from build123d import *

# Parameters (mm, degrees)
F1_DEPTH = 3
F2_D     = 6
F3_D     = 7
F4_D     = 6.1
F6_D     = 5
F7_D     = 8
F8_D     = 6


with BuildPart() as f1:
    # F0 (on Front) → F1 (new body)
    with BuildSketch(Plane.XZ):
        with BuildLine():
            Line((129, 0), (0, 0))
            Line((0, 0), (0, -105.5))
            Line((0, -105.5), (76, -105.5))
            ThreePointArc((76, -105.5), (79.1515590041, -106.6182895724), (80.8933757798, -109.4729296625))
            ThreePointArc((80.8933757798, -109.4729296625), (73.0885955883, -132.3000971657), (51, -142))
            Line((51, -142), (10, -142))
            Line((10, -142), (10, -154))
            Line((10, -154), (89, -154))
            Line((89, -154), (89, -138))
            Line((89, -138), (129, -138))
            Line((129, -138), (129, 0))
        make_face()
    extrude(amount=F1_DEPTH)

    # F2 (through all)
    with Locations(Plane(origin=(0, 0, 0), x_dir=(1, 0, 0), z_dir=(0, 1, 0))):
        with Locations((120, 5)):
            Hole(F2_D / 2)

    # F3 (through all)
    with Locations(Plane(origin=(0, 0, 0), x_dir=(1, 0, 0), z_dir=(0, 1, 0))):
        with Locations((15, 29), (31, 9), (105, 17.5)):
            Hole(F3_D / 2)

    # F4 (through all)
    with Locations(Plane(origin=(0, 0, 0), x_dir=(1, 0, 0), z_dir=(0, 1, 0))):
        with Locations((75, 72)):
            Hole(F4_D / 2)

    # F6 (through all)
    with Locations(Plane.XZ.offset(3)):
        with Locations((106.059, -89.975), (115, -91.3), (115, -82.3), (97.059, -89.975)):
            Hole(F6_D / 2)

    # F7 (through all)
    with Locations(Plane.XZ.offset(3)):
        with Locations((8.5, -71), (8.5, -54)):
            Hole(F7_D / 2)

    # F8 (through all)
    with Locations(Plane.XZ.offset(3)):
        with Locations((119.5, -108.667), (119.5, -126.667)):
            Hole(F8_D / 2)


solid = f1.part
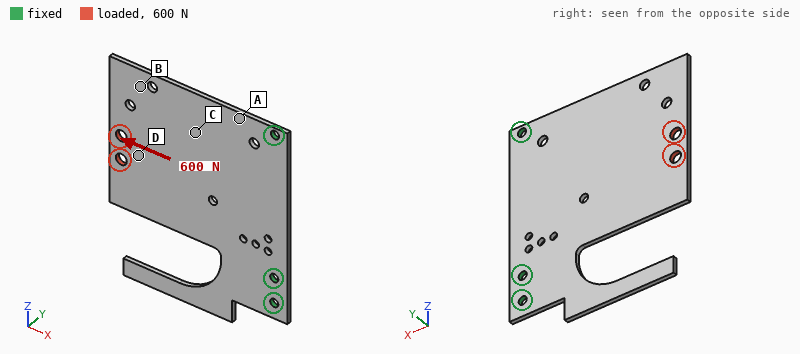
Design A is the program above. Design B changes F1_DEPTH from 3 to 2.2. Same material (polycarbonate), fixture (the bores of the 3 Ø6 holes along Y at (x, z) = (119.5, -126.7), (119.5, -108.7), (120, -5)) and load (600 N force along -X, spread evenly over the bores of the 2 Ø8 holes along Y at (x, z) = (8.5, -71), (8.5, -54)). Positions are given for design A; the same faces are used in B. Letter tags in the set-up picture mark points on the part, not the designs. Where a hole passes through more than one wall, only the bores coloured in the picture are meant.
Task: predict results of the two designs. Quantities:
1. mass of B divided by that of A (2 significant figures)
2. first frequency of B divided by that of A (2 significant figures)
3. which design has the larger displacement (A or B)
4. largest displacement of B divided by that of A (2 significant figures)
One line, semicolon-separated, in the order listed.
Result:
0.73; 0.74; B; 1.4
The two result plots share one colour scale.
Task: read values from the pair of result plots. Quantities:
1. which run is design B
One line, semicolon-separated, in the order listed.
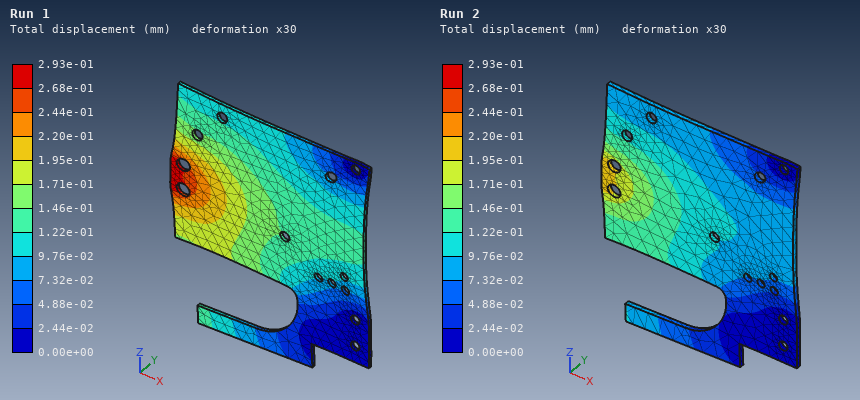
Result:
Run 1
